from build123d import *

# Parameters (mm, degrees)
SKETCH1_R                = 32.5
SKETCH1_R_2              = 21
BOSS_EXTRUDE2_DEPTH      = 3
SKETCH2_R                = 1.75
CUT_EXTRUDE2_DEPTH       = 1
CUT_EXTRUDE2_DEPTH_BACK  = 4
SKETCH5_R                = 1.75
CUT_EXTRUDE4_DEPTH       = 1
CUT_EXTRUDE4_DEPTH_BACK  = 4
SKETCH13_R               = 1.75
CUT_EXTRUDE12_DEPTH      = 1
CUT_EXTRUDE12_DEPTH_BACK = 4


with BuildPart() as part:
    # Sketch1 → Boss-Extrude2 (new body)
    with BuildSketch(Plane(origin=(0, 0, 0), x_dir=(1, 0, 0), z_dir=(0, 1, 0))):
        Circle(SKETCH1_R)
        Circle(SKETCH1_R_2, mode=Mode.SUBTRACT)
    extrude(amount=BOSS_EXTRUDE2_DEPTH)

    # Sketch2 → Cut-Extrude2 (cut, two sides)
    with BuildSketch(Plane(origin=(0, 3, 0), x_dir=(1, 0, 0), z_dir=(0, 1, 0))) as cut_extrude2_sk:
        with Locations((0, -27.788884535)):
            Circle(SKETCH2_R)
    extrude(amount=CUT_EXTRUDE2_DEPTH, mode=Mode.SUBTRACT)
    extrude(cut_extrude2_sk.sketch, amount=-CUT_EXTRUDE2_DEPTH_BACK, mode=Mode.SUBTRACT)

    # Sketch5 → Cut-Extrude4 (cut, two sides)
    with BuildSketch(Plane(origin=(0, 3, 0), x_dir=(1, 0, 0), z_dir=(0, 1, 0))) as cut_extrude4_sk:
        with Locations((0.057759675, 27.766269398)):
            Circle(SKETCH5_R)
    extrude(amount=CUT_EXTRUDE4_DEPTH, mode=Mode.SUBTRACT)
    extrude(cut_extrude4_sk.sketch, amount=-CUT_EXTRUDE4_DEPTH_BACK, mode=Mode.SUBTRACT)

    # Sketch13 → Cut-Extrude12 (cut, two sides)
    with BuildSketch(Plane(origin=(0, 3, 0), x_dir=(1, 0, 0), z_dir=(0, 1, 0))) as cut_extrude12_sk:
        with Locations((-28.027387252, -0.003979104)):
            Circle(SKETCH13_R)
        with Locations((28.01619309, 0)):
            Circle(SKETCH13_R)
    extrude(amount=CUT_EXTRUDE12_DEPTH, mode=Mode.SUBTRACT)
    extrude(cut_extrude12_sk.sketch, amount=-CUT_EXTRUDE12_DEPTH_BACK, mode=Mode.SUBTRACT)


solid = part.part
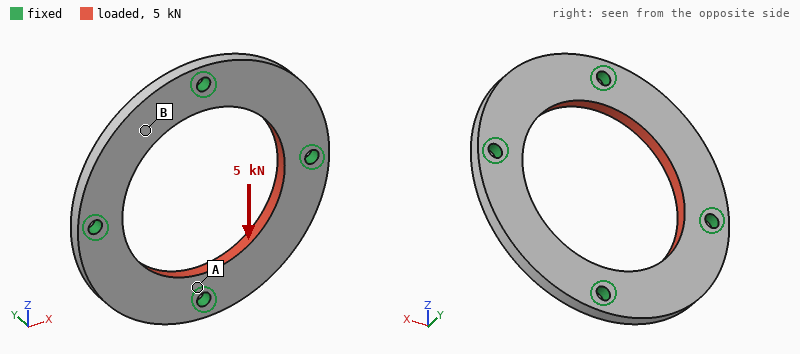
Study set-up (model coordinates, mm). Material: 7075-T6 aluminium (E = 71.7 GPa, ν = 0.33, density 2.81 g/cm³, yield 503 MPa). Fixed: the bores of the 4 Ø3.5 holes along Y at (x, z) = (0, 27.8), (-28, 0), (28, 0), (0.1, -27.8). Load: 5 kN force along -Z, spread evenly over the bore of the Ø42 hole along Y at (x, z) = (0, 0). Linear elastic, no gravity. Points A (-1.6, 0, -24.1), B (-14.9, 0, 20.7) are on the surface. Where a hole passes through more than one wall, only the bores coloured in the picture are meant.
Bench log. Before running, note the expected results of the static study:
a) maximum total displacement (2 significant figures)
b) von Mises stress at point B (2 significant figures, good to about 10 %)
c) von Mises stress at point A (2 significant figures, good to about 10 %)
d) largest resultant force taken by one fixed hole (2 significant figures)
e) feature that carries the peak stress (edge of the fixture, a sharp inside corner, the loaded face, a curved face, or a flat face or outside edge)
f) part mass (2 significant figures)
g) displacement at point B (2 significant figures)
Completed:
11 µm
14 MPa
36 MPa
1.6 kN
edge of the fixture
16 g
10 µm
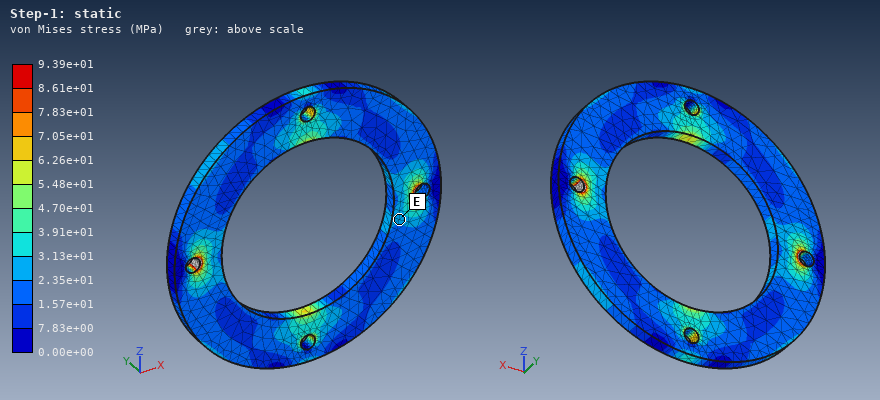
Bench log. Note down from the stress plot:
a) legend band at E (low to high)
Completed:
2.35e+01 to 3.13e+01 MPa
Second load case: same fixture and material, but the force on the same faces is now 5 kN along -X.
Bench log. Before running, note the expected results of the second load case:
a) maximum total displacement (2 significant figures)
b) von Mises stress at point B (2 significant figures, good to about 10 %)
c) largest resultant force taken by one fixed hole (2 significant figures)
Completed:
11 µm
13 MPa
1.6 kN
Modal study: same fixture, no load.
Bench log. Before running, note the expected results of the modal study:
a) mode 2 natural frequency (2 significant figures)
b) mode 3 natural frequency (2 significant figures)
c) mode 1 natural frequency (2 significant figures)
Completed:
8100 Hz
8100 Hz
7800 Hz
